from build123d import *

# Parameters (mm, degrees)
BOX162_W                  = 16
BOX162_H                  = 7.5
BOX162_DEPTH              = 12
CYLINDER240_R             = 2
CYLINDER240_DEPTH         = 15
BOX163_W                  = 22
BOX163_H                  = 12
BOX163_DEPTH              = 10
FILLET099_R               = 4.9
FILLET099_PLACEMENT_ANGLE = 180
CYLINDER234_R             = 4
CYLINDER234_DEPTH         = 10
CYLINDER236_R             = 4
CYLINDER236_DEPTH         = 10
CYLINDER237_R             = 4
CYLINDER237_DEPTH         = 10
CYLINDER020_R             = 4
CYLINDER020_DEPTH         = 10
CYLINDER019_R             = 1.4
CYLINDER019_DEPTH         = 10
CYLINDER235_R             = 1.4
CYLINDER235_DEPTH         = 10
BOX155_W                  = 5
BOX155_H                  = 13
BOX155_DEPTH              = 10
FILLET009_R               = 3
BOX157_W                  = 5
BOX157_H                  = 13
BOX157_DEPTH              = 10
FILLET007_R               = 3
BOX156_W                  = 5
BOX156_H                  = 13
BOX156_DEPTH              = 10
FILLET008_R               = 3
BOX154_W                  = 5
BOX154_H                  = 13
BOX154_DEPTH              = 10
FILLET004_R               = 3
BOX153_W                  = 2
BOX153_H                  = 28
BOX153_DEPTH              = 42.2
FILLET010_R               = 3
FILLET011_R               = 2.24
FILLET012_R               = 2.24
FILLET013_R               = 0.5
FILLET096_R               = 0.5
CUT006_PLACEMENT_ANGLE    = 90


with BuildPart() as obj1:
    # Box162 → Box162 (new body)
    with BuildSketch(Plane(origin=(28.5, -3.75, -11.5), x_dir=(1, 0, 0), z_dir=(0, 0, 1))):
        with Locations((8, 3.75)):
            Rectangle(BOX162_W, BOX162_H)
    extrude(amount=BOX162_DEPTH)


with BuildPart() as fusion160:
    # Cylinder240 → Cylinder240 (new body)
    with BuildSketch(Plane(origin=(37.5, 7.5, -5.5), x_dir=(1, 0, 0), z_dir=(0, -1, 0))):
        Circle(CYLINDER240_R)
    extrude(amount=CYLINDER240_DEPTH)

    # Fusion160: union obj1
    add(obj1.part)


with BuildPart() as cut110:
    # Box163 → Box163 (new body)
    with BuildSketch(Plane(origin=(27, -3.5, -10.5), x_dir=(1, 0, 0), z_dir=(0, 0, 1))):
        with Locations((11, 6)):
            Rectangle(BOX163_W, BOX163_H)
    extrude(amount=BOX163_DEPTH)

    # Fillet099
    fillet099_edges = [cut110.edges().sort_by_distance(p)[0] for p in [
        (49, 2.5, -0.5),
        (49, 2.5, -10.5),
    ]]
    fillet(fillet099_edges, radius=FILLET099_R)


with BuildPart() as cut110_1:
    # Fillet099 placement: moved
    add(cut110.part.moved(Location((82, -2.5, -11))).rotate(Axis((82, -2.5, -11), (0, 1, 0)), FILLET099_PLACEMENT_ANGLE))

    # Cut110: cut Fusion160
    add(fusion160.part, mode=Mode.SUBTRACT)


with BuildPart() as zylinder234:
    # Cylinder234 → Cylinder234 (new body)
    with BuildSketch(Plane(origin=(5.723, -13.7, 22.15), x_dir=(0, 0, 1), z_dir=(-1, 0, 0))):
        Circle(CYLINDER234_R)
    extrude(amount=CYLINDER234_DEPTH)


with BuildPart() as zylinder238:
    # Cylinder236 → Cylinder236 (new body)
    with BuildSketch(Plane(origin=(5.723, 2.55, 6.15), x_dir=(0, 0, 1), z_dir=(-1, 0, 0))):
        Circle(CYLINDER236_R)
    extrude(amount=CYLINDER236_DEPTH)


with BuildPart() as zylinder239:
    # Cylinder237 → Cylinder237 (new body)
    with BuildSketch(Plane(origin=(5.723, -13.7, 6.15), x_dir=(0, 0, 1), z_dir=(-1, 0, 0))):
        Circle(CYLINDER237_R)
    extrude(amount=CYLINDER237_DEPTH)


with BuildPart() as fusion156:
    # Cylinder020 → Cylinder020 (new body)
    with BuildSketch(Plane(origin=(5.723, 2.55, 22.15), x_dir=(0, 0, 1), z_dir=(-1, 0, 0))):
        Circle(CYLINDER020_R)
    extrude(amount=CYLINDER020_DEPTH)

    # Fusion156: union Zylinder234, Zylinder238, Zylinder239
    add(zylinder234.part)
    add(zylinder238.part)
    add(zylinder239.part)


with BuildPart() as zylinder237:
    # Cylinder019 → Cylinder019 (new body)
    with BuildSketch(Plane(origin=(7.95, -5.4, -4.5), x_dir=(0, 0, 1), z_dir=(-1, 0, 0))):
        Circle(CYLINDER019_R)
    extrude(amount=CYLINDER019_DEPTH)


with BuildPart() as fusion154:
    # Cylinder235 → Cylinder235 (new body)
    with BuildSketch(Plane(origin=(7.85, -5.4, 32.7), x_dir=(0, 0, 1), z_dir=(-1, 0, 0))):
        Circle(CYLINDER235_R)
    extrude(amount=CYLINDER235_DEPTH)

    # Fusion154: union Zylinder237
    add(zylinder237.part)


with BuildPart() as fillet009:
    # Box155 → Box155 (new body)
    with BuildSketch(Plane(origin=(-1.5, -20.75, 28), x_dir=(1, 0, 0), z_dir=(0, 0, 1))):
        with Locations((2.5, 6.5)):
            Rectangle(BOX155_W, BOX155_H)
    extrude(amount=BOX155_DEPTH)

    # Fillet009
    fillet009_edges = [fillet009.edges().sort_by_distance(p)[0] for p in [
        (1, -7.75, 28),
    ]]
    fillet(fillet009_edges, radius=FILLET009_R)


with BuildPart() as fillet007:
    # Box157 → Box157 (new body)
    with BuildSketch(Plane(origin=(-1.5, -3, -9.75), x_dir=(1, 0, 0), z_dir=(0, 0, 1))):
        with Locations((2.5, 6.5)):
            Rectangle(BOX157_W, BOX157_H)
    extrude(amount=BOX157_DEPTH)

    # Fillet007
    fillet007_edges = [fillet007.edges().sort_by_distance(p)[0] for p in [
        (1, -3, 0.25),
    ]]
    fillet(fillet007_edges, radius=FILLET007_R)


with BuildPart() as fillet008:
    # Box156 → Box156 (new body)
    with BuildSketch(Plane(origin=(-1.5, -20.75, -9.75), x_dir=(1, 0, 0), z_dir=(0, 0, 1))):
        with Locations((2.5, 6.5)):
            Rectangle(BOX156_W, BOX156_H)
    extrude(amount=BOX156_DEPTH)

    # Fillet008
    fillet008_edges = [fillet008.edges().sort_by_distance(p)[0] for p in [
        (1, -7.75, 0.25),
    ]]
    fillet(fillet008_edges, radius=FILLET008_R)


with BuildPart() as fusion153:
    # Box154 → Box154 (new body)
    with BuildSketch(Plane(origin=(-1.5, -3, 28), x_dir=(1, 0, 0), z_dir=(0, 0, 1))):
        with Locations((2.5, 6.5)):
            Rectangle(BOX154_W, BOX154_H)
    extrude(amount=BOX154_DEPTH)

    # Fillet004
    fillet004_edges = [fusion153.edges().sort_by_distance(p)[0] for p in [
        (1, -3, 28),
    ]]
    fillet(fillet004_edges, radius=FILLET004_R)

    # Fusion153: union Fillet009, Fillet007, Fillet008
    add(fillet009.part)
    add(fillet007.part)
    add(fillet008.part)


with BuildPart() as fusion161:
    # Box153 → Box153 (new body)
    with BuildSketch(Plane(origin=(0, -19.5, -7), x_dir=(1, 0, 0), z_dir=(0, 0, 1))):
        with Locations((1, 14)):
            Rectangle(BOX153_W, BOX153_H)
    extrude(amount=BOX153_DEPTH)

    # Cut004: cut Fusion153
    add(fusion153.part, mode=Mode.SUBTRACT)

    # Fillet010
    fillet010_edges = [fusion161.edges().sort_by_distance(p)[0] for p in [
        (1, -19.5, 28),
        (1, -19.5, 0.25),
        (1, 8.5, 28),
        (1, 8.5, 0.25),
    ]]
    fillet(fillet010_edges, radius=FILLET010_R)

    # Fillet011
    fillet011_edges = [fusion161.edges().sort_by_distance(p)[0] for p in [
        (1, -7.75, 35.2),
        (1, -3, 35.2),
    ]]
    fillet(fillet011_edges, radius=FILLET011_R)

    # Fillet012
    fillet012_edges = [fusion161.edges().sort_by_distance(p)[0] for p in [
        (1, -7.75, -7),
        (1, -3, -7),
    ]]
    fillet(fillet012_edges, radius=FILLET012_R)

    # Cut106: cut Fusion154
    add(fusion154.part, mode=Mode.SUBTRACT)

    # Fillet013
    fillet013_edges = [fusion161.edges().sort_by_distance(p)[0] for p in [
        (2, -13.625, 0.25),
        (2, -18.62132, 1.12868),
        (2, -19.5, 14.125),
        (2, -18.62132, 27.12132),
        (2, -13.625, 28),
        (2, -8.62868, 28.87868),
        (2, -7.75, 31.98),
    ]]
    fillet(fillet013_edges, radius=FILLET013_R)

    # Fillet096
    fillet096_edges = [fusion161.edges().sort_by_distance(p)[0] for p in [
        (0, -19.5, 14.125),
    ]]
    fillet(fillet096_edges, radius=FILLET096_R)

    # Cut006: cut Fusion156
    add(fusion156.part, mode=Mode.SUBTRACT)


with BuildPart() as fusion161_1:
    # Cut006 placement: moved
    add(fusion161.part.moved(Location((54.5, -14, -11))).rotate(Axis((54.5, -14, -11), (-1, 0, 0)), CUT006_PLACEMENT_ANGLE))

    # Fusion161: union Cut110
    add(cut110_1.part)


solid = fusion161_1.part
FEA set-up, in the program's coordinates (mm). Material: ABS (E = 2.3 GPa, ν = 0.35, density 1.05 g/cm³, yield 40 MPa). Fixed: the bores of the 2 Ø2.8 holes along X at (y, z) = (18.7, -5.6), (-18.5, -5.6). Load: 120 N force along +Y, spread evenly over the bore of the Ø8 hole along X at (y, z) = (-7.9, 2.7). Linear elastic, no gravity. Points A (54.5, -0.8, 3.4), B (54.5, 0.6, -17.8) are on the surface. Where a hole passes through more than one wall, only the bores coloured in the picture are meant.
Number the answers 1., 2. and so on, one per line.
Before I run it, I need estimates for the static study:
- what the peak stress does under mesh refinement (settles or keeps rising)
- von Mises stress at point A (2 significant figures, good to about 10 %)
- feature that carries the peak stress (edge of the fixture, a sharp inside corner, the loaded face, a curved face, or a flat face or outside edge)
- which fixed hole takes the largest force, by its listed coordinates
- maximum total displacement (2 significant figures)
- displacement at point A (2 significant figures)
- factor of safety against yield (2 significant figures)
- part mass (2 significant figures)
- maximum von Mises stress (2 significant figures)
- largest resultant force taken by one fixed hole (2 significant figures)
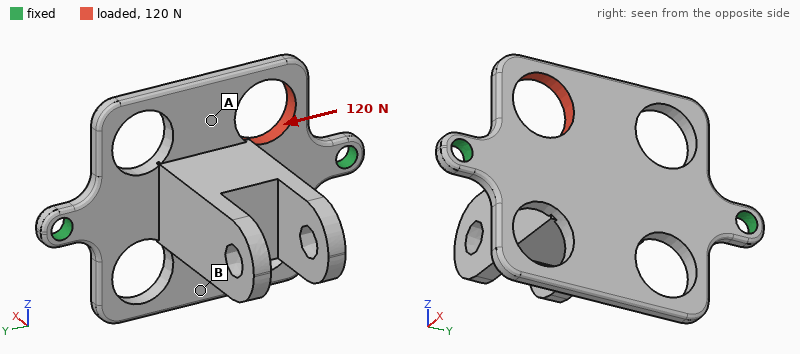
1. settles
2. 5.3 MPa
3. a curved face
4. (-18.5, -5.6)
5. 0.13 mm
6. 0.070 mm
7. 1.8
8. 3.0 g
9. 22 MPa
10. 75 N
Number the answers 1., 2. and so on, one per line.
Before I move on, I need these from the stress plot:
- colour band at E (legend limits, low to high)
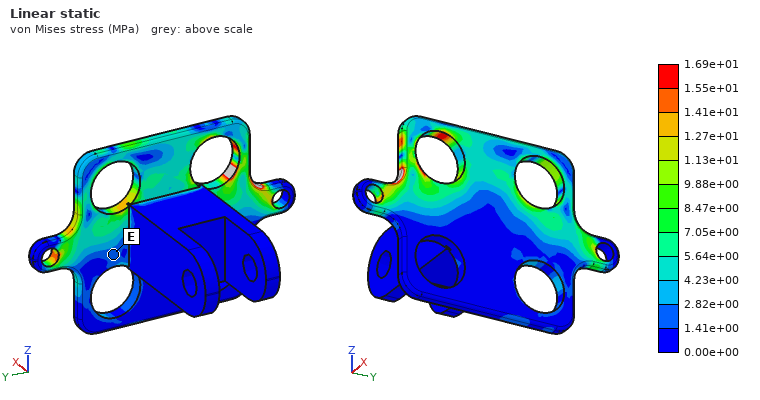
1. 1.41e+00 to 2.82e+00 MPa
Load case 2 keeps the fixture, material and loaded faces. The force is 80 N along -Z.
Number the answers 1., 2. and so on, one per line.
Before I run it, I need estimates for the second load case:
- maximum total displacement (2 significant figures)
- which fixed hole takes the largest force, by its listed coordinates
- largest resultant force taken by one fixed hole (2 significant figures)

1. 0.10 mm
2. (-18.5, -5.6)
3. 60 N
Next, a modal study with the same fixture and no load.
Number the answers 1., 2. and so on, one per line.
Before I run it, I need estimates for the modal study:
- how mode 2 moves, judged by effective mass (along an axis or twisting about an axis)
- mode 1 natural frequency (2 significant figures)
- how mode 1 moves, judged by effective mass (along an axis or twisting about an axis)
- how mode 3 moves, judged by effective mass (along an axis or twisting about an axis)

1. along X
2. 540 Hz
3. along Z
4. along Y
